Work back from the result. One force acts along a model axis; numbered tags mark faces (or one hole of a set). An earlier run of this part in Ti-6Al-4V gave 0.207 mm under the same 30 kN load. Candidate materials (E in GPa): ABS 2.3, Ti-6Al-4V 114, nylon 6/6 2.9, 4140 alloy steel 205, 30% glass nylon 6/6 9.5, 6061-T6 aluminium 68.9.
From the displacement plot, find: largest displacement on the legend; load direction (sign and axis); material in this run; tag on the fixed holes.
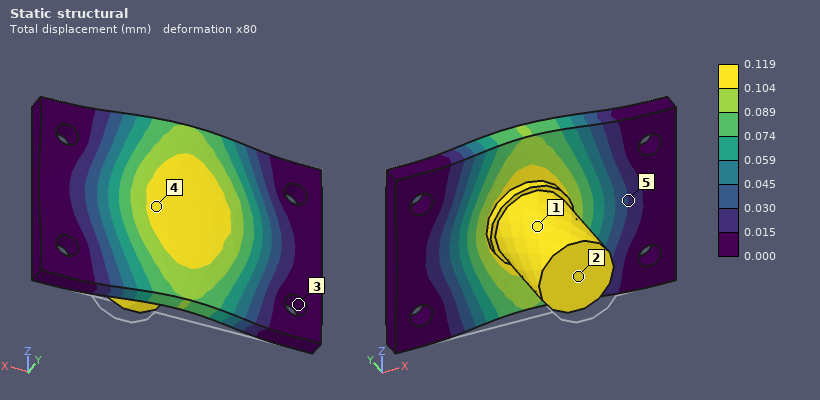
0.119 mm
+Y
4140 alloy steel
3
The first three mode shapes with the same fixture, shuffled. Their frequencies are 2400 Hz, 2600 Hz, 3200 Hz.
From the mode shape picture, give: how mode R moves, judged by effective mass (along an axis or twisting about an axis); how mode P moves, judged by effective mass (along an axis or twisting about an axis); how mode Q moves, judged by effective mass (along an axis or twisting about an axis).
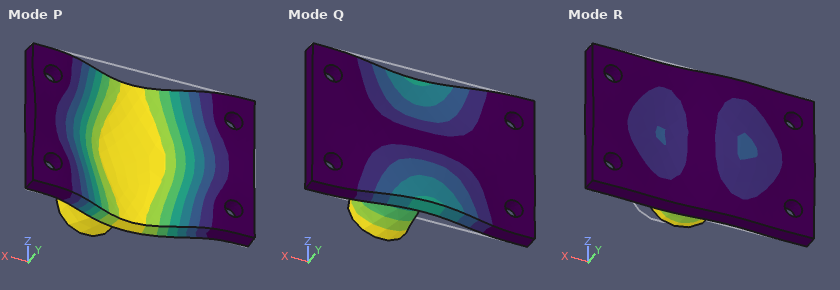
along X
along Y
along Z
